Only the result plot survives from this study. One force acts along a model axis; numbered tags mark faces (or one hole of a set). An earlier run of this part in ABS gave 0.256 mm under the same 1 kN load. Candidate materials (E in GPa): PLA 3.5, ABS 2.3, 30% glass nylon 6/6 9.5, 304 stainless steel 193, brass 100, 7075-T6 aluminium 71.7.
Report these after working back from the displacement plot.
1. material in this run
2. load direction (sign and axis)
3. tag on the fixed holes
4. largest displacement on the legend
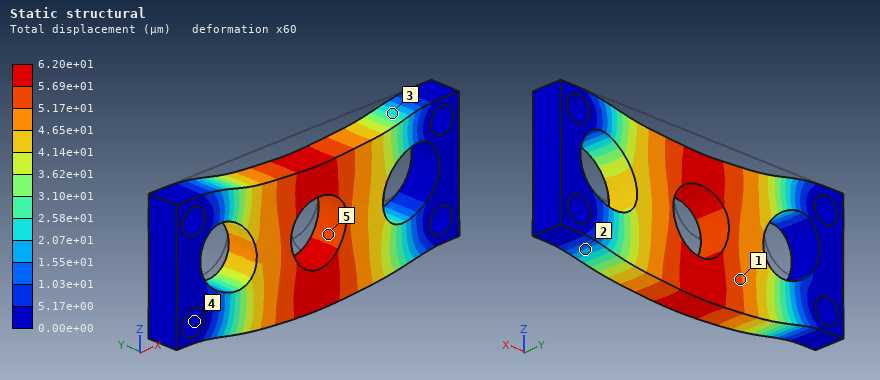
30% glass nylon 6/6
-Z
4
6.20e+01 µm
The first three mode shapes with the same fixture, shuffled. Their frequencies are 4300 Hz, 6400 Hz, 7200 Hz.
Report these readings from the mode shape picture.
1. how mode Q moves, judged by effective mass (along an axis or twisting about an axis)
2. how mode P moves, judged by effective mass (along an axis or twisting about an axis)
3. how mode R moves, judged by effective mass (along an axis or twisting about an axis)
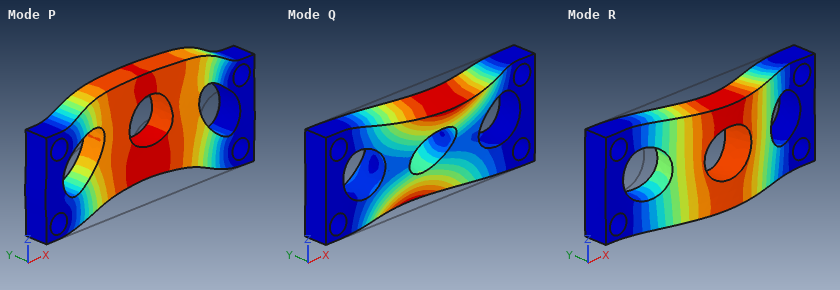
twisting about X
along Z
along Y
